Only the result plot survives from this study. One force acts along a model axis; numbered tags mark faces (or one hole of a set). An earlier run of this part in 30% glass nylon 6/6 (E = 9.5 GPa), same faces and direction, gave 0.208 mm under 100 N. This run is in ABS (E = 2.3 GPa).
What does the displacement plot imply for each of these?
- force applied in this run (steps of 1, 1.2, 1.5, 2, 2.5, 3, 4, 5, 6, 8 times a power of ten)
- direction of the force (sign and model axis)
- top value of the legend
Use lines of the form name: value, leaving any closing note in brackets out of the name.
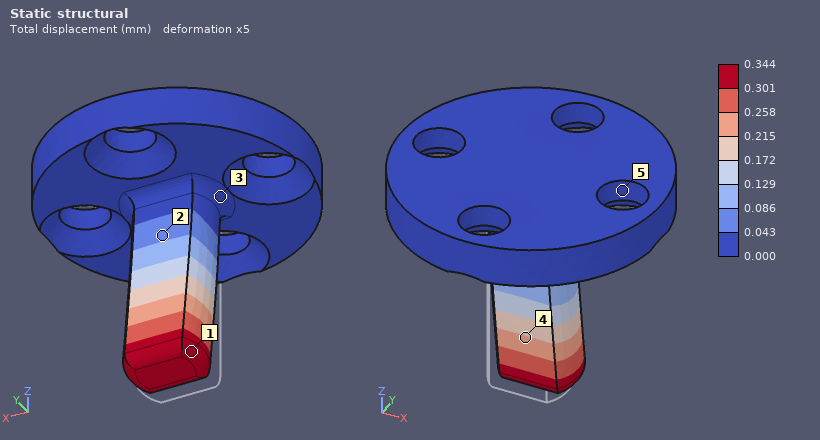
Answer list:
force applied in this run: 40 N
direction of the force: +Y
top value of the legend: 0.344 mm
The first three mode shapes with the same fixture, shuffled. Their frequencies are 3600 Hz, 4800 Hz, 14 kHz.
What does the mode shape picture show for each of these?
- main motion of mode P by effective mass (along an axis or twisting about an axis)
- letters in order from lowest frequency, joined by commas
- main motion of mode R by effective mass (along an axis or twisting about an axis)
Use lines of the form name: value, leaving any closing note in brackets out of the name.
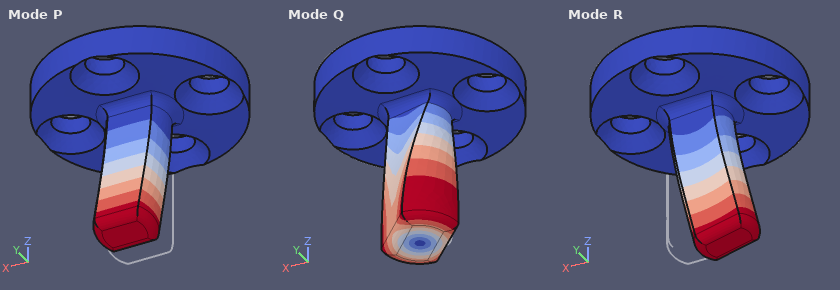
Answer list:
main motion of mode P by effective mass: along Y
letters in order from lowest frequency, joined by commas: P, R, Q
main motion of mode R by effective mass: along X
